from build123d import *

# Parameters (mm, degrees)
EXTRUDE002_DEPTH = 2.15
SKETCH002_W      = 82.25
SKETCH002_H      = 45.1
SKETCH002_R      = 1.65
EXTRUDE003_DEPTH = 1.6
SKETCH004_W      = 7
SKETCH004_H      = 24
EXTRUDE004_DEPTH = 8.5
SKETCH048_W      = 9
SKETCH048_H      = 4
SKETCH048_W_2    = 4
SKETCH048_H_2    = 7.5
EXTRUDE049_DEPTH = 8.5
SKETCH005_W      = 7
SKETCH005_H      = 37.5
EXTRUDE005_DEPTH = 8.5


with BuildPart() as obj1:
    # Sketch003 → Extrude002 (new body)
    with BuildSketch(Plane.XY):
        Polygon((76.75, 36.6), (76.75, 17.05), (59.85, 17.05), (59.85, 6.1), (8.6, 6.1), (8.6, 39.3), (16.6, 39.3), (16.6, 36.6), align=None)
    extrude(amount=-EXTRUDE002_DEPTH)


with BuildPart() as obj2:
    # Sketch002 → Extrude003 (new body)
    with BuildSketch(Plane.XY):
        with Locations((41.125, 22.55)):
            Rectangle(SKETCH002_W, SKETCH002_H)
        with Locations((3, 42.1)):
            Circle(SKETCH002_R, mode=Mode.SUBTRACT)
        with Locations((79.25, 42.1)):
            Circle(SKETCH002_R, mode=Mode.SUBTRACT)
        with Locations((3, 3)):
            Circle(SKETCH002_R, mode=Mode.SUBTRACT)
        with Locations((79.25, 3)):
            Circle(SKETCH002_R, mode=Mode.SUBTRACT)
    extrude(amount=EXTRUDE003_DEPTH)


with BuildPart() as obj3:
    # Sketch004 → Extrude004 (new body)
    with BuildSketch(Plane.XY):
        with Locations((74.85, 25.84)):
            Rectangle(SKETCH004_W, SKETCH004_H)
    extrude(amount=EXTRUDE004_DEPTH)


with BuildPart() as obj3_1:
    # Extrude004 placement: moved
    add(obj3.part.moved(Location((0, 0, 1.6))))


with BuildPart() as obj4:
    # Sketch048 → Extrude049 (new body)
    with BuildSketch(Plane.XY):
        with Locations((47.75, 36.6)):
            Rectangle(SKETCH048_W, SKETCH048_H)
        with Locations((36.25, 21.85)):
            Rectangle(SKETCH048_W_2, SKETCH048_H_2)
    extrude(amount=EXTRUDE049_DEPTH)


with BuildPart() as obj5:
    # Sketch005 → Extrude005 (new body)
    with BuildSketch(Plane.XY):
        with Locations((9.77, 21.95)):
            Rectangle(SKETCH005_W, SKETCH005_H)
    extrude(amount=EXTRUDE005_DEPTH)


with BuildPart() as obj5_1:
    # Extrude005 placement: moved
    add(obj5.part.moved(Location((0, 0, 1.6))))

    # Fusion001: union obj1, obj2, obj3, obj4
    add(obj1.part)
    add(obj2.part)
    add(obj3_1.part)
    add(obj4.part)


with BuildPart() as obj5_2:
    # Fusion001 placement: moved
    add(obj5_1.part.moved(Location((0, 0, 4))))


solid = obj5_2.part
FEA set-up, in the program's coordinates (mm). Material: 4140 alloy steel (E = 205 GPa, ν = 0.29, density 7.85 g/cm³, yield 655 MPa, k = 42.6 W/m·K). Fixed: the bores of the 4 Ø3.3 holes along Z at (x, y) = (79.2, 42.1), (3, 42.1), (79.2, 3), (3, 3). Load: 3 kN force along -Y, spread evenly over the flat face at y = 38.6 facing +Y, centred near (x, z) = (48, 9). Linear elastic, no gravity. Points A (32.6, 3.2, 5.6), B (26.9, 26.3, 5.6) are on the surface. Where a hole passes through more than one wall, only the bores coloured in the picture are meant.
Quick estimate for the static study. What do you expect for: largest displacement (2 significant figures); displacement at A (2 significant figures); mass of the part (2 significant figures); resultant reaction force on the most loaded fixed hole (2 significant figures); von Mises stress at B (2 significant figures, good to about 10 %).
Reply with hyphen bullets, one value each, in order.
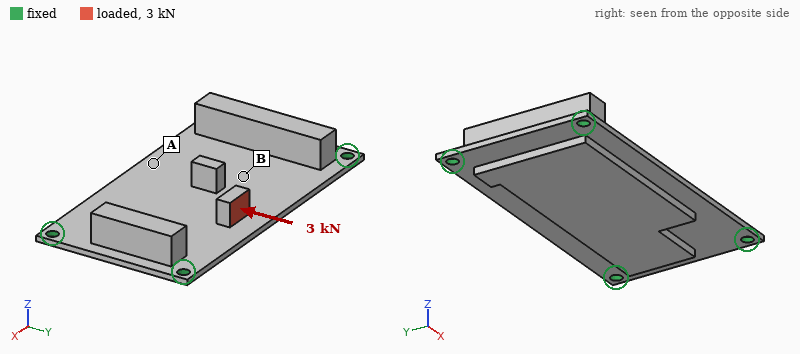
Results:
- 0.18 mm
- 0.038 mm
- 110 g
- 1.1 kN
- 110 MPa
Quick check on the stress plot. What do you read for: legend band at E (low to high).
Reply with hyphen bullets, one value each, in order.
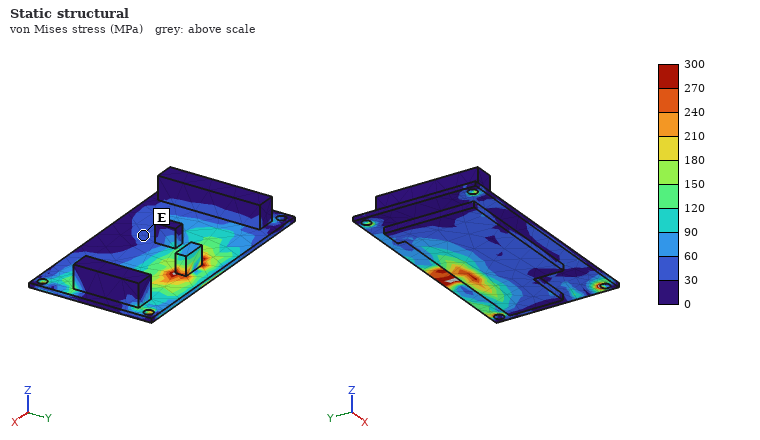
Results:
- 30 to 60 MPa
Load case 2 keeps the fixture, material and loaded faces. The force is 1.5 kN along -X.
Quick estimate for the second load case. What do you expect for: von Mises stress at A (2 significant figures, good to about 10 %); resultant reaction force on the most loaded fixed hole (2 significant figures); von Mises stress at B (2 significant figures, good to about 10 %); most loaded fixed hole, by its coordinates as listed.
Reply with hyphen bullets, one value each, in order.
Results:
- 13 MPa
- 570 N
- 30 MPa
- (79.2, 42.1)
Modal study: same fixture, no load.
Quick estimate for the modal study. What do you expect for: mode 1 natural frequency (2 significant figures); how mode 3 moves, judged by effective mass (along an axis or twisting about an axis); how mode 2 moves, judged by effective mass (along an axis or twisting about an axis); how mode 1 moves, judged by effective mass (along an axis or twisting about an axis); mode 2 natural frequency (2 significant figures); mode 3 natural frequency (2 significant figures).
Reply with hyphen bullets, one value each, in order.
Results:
- 1800 Hz
- twisting about Y
- twisting about X
- along Z
- 4300 Hz
- 5100 Hz
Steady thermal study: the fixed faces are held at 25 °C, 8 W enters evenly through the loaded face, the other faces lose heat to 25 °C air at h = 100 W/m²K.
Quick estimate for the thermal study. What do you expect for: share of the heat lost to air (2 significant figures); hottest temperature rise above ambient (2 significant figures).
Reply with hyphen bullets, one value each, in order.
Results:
- 81 %
- 50 K
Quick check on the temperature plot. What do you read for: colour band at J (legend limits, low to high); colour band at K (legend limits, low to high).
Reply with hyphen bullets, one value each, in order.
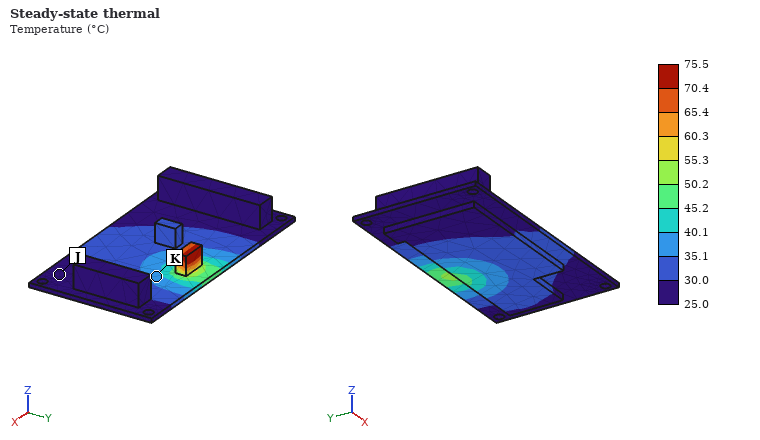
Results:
- 25.0 to 30.0 °C
- 35.1 to 40.1 °C
